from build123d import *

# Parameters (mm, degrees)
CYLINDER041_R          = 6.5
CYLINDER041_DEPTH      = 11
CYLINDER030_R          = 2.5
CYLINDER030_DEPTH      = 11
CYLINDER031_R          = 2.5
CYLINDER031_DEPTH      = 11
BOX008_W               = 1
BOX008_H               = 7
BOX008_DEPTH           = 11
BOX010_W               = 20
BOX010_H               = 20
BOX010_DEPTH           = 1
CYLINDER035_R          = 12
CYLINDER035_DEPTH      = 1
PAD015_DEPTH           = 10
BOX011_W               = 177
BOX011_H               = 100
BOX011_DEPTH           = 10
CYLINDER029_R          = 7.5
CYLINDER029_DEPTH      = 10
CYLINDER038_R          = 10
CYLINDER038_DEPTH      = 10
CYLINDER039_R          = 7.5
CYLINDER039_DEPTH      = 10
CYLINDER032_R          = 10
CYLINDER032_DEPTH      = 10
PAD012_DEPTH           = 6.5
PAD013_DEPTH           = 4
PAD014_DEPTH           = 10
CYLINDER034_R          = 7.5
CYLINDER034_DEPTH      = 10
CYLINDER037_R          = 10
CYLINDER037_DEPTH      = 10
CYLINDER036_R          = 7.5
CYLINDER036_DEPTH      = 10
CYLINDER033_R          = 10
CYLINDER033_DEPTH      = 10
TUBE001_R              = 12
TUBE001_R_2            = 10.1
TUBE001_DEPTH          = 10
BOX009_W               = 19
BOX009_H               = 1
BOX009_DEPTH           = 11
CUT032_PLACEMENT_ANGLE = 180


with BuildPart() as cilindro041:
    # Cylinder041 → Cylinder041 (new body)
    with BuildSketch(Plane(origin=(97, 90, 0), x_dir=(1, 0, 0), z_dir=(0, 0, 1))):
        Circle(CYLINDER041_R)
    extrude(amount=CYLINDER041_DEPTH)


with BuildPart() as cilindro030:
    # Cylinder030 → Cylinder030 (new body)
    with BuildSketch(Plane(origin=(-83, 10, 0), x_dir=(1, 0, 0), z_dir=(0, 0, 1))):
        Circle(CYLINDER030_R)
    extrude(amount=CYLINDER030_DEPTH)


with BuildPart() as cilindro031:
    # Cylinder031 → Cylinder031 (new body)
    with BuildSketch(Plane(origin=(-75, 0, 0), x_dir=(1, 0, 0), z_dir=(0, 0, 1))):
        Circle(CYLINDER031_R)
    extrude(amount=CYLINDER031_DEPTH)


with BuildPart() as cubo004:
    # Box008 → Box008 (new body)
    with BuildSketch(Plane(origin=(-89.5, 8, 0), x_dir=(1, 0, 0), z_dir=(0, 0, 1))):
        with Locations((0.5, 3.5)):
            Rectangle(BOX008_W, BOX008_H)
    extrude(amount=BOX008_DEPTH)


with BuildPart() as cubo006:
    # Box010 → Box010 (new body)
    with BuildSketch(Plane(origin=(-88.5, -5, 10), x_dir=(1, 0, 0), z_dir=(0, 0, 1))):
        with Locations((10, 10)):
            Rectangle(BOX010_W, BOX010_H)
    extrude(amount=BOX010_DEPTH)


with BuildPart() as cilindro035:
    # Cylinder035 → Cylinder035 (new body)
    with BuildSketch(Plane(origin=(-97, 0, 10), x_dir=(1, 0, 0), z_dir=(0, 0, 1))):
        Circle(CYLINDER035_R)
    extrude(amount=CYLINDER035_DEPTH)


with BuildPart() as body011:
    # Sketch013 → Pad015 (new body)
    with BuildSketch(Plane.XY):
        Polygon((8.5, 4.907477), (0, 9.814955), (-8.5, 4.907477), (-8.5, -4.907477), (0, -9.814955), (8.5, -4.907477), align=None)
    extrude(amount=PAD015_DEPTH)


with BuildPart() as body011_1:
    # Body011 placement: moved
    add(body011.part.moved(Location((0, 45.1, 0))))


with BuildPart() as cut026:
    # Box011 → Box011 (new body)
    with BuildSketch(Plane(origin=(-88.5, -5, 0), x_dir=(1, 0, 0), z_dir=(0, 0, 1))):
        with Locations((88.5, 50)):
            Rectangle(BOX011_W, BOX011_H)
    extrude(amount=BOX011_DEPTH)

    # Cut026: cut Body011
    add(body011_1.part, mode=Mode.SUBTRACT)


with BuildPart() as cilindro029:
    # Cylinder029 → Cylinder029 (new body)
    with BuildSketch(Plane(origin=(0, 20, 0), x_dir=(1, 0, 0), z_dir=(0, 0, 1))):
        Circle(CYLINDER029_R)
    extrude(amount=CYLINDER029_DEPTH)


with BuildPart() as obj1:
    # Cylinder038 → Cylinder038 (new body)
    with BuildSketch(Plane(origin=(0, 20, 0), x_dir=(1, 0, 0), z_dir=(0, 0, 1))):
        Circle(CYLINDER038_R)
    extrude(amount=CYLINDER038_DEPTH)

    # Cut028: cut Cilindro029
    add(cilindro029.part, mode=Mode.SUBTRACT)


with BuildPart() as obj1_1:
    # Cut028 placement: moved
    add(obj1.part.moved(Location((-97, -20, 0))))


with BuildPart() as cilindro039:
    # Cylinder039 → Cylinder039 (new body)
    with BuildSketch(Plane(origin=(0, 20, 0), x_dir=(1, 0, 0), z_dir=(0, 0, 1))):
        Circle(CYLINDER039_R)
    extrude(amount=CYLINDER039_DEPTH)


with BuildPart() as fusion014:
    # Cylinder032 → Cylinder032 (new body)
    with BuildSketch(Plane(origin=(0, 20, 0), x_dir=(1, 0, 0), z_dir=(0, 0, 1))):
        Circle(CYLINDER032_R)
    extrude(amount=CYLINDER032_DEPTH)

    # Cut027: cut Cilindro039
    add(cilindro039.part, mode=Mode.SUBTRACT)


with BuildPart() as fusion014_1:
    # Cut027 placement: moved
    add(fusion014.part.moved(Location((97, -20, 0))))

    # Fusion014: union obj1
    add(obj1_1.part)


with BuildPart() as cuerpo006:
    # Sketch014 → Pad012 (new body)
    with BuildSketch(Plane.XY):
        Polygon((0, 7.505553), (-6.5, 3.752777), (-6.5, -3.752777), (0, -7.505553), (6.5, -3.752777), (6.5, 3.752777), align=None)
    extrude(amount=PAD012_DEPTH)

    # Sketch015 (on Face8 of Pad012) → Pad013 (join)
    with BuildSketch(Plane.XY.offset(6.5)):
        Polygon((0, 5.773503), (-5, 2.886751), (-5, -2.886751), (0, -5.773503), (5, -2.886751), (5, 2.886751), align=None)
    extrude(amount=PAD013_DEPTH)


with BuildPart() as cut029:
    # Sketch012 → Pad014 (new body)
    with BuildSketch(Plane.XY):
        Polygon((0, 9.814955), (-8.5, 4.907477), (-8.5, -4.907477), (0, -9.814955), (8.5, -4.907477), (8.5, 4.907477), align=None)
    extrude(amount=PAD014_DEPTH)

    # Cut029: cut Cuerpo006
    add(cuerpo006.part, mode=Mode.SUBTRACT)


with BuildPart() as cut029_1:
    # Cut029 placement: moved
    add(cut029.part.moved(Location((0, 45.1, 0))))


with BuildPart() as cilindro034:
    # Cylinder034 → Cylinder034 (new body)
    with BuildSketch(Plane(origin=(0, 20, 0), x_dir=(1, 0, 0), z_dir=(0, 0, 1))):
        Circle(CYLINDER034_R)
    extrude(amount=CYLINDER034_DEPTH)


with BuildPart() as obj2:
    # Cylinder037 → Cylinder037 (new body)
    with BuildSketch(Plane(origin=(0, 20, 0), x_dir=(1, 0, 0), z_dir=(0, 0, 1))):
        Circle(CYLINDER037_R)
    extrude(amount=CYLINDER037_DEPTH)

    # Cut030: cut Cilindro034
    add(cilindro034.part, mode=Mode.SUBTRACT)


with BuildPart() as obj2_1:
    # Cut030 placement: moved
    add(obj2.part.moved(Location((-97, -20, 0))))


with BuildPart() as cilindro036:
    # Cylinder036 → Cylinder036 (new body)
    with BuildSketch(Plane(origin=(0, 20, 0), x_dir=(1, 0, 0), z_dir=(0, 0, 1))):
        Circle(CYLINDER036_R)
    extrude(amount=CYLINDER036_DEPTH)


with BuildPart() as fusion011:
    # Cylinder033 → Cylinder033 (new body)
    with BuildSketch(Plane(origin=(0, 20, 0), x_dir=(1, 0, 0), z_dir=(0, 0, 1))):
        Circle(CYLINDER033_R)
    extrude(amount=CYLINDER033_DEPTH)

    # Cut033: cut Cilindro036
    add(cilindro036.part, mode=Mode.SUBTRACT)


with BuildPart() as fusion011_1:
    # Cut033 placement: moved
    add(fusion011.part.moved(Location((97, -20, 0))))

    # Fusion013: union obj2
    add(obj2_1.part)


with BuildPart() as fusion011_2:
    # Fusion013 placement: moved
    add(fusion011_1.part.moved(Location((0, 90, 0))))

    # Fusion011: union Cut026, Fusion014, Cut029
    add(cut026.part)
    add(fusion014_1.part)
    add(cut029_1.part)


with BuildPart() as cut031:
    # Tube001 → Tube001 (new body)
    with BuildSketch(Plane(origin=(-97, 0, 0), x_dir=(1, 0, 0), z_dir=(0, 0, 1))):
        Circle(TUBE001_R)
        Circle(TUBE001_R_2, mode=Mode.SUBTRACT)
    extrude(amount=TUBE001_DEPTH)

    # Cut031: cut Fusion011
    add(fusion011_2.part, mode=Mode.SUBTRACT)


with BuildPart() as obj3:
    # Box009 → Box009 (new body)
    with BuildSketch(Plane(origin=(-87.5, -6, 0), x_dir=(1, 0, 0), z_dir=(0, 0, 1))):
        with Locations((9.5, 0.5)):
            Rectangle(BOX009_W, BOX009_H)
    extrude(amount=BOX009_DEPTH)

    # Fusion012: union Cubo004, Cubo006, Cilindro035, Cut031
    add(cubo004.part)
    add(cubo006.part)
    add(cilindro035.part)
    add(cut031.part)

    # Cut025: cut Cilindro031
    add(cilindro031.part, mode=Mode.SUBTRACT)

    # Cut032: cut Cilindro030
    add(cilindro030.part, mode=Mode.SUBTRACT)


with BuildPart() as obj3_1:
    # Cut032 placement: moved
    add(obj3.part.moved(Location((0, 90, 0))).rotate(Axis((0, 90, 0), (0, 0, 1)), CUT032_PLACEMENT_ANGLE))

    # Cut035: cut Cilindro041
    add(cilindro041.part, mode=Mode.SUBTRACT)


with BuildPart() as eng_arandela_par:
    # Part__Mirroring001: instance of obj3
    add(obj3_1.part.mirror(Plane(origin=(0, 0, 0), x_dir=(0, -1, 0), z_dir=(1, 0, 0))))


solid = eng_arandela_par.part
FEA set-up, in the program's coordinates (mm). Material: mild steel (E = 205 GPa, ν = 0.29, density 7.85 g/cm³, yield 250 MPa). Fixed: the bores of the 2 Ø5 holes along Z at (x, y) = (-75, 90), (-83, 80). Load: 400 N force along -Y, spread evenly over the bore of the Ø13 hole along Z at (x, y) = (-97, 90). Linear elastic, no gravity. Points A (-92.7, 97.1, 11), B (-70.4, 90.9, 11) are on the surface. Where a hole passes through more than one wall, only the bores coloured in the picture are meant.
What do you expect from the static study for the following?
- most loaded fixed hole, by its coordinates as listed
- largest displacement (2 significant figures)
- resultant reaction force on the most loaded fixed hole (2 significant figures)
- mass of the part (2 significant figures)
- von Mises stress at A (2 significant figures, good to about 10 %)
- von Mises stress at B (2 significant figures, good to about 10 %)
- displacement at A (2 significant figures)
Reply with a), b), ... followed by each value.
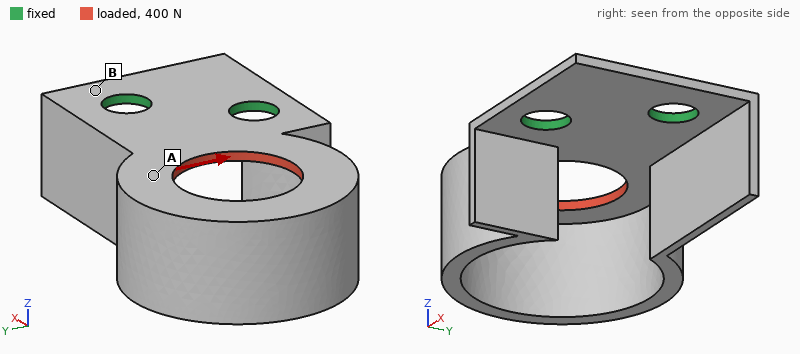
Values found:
a) (-83, 80)
b) 31 µm
c) 570 N
d) 16 g
e) 58 MPa
f) 15 MPa
g) 13 µm
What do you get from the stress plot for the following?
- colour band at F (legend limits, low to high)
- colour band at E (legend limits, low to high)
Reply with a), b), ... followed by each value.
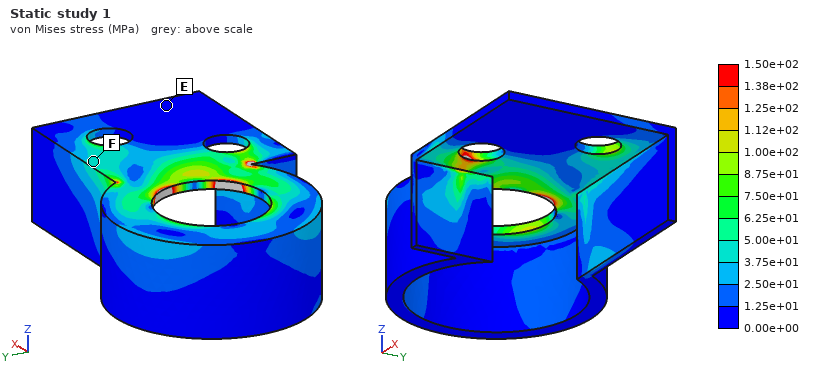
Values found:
a) 3.75e+01 to 5.00e+01 MPa
b) 0.00e+00 to 1.25e+01 MPa
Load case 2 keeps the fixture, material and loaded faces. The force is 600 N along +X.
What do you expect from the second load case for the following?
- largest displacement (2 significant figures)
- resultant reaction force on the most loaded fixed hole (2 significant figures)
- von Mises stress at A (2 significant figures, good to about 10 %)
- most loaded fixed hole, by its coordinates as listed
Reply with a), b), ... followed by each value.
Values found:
a) 17 µm
b) 440 N
c) 58 MPa
d) (-75, 90)
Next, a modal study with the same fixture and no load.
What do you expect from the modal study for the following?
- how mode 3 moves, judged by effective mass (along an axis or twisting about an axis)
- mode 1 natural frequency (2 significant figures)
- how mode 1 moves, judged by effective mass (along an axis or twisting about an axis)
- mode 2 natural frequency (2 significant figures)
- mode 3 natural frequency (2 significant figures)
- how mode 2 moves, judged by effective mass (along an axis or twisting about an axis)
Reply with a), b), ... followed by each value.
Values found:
a) along Y
b) 1100 Hz
c) along Z
d) 2700 Hz
e) 5700 Hz
f) along Y
